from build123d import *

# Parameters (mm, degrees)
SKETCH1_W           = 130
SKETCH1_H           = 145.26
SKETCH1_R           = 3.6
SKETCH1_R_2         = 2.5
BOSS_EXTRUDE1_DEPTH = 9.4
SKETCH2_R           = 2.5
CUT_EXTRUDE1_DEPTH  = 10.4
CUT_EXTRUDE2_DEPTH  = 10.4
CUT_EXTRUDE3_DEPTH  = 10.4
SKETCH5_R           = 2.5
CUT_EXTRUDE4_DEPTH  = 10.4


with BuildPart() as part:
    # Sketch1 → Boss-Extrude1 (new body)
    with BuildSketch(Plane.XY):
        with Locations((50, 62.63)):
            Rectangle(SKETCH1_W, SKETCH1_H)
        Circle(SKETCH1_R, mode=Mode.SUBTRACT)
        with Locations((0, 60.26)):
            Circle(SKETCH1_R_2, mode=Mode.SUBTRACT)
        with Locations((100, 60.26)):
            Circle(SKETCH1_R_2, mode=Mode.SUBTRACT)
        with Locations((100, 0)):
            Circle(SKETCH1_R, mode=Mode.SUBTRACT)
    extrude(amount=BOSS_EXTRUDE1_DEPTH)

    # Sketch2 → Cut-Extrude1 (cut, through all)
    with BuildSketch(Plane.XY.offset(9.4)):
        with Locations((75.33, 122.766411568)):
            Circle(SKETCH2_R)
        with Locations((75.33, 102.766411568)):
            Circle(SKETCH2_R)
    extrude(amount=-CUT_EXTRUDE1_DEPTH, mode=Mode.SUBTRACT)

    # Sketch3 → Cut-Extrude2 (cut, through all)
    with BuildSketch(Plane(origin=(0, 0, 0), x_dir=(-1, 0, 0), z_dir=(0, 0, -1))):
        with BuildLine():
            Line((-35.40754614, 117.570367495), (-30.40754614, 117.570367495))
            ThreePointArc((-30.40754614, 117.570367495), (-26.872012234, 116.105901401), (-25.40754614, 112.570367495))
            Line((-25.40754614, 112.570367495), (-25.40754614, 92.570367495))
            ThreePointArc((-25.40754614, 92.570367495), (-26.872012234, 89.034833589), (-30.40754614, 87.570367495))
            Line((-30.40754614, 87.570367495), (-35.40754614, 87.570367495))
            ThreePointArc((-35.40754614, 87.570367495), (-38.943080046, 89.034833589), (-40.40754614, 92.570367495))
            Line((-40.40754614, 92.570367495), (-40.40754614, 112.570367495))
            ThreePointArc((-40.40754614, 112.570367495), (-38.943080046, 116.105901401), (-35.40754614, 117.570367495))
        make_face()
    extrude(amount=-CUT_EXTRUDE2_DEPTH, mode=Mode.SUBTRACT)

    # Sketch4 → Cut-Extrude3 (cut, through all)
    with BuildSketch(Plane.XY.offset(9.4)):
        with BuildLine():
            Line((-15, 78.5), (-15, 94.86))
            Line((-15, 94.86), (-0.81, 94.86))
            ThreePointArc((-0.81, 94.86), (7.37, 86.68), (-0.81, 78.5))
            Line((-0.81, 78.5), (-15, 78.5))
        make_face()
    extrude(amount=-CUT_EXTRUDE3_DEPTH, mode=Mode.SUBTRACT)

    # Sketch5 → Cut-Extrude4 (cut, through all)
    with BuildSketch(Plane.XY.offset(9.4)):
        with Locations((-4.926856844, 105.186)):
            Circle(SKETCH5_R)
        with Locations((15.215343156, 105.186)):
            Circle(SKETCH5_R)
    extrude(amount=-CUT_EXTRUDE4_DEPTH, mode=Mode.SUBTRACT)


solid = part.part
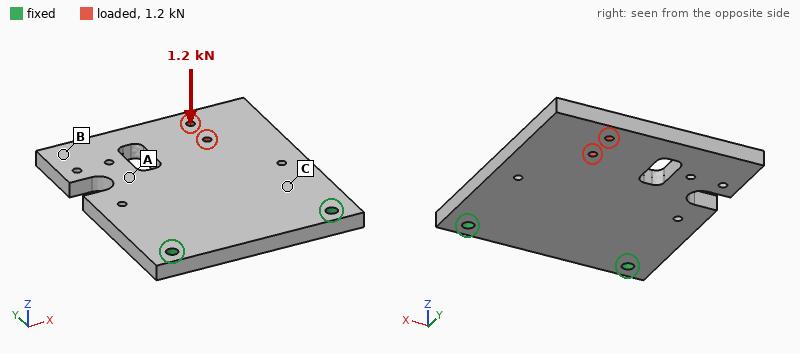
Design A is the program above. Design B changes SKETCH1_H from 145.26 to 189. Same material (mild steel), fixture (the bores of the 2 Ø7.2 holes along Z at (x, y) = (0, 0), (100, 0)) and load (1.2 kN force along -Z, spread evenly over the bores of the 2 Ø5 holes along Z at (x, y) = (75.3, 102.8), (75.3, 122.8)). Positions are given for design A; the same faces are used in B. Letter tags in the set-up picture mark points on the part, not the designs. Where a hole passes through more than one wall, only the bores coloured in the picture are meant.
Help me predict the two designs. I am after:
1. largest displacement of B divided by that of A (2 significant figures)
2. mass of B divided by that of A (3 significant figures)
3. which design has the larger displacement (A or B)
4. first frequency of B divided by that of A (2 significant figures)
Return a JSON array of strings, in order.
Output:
["1.1", "1.32", "B", "0.76"]
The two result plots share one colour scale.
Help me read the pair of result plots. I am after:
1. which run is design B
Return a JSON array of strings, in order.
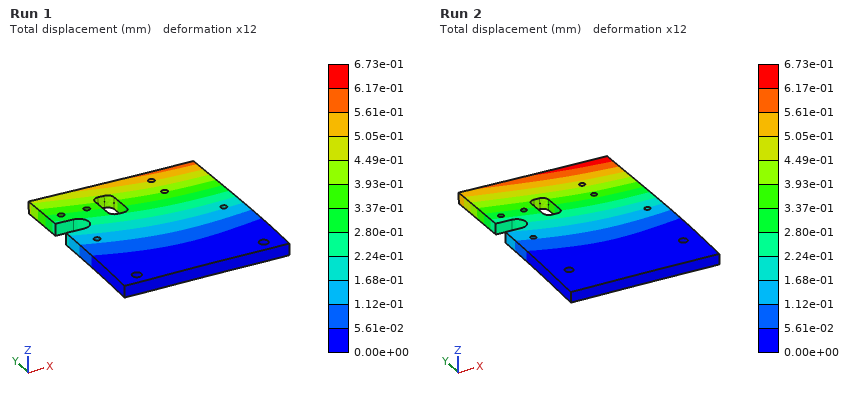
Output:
["Run 2"]
